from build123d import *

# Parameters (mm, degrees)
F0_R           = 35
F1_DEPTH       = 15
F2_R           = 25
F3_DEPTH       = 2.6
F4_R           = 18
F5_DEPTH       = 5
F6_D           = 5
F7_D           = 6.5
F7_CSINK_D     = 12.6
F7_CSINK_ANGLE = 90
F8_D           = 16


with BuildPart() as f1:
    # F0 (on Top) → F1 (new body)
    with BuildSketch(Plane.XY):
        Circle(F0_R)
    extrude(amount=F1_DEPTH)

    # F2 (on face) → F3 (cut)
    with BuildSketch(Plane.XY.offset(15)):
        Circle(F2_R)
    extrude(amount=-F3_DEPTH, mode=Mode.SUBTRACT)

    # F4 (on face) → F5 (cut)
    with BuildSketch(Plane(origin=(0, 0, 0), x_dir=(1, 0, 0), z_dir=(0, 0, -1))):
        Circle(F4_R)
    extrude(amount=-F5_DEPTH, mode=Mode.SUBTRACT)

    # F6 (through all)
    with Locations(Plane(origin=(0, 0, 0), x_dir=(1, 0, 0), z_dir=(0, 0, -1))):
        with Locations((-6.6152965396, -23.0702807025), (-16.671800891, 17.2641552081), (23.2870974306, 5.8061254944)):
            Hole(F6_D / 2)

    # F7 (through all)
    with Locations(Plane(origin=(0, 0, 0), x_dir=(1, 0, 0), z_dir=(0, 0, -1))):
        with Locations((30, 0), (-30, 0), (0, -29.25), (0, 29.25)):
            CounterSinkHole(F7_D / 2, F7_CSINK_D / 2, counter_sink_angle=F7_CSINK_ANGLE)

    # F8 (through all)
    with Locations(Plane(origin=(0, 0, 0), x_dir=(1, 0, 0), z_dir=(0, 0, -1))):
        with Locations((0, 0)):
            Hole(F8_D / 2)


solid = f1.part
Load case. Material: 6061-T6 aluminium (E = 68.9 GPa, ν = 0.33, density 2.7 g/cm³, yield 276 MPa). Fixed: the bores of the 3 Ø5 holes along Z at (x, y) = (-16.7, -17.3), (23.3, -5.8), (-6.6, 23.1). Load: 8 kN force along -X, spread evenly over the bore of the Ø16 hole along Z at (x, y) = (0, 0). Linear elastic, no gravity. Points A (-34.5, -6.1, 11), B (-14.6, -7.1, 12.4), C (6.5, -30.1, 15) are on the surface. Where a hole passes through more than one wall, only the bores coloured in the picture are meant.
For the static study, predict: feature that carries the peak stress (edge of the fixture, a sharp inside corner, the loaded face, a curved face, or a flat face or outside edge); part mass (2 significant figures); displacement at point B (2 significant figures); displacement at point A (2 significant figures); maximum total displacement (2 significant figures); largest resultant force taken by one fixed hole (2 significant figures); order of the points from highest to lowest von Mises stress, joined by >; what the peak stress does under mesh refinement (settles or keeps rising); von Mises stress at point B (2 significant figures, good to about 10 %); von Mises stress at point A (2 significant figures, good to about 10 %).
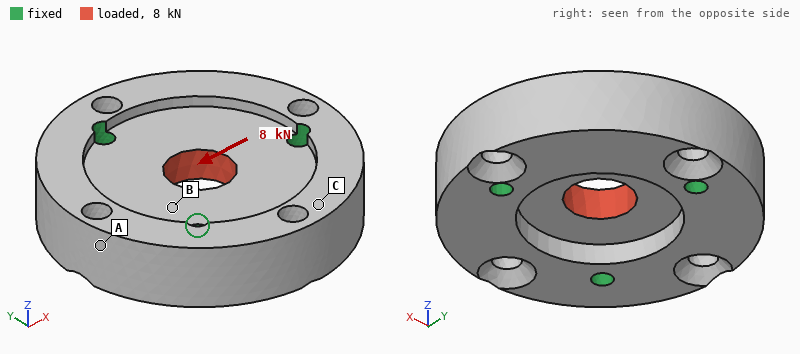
edge of the fixture
120 g
4.3 µm
3.7 µm
8.1 µm
2.7 kN
B > A > C
keeps rising
17 MPa
11 MPa
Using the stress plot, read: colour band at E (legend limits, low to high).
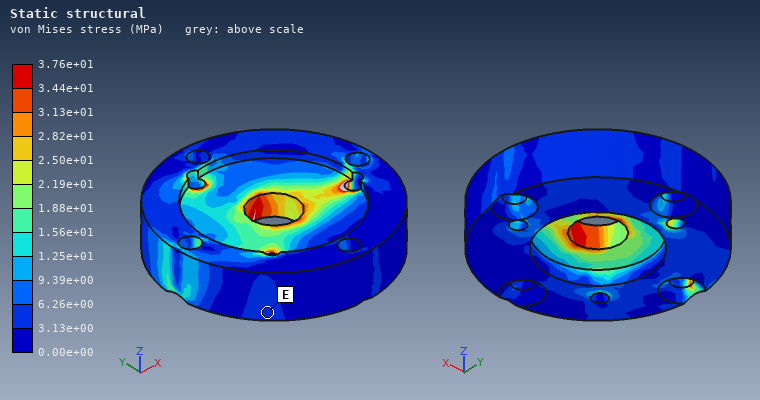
3.13e+00 to 6.26e+00 MPa
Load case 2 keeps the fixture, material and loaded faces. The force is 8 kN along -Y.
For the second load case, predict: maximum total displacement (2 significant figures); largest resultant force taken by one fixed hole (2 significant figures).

8.1 µm
2.7 kN
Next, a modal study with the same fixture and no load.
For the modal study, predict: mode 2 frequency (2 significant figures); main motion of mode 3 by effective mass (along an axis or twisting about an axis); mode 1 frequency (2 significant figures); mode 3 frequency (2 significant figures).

14 kHz
along Z
12 kHz
16 kHz
